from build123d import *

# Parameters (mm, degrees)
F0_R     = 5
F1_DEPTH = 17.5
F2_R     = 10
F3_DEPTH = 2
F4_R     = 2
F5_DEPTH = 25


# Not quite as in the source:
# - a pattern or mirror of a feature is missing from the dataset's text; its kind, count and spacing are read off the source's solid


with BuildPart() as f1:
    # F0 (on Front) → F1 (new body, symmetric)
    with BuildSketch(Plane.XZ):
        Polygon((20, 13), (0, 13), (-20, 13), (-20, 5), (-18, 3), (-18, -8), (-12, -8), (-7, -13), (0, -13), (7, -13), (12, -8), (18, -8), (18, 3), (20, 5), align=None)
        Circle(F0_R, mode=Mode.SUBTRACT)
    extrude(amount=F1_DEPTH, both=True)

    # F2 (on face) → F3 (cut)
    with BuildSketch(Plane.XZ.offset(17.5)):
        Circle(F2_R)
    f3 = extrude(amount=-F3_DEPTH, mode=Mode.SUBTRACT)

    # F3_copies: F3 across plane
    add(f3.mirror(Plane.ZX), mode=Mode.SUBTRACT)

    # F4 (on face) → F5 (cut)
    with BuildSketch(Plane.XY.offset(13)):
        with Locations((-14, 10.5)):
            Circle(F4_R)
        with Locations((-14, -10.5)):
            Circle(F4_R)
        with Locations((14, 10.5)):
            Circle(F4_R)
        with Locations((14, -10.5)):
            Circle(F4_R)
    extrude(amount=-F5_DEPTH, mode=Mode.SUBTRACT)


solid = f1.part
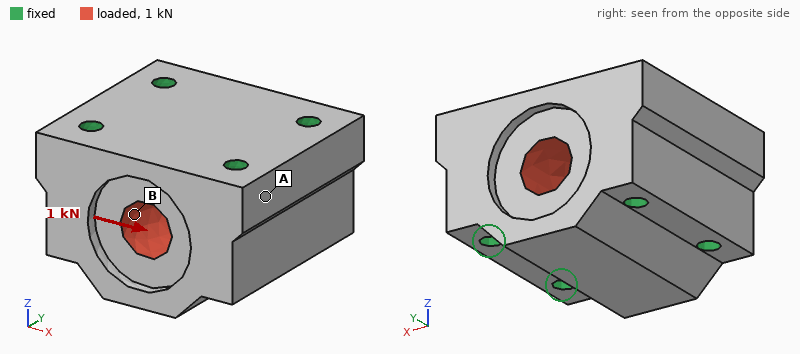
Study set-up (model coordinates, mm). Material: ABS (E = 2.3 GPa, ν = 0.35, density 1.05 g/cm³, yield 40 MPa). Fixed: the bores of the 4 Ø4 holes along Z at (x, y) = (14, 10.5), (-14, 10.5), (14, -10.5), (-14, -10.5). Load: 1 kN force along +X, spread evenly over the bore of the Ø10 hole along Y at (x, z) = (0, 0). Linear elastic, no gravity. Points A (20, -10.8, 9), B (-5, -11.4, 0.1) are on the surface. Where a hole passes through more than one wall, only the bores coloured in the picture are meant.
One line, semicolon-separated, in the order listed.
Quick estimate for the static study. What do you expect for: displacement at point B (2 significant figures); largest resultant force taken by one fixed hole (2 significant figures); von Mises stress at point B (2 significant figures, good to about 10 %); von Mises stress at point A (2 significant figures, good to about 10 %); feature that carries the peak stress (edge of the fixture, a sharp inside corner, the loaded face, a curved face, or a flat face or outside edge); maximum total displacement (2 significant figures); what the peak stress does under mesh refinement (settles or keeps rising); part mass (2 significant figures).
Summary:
4.0 µm; 260 N; 1.1 MPa; 0.40 MPa; edge of the fixture; 7.6 µm; keeps rising; 28 g
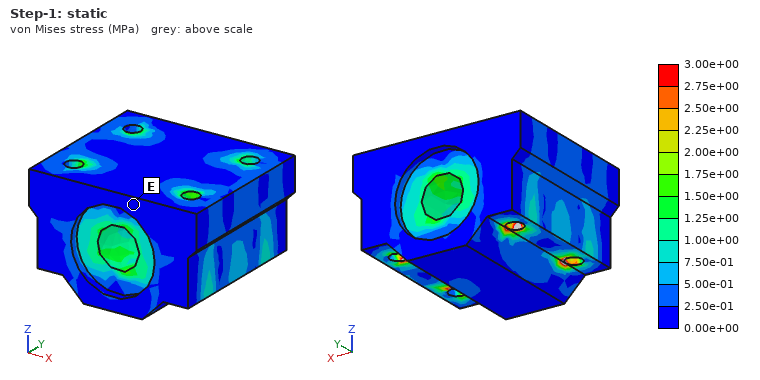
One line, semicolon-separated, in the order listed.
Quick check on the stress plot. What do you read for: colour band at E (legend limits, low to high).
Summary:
0.00e+00 to 2.50e-01 MPa
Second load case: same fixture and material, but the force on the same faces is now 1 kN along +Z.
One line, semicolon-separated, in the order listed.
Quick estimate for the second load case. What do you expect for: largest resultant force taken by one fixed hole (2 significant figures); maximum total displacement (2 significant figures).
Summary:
250 N; 14 µm
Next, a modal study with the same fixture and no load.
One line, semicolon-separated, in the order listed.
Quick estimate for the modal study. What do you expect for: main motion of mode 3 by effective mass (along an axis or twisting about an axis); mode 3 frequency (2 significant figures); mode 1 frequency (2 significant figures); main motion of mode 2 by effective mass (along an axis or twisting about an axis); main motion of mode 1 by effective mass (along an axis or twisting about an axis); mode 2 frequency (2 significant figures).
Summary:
along Y; 16 kHz; 13 kHz; along Z; along Y; 14 kHz
